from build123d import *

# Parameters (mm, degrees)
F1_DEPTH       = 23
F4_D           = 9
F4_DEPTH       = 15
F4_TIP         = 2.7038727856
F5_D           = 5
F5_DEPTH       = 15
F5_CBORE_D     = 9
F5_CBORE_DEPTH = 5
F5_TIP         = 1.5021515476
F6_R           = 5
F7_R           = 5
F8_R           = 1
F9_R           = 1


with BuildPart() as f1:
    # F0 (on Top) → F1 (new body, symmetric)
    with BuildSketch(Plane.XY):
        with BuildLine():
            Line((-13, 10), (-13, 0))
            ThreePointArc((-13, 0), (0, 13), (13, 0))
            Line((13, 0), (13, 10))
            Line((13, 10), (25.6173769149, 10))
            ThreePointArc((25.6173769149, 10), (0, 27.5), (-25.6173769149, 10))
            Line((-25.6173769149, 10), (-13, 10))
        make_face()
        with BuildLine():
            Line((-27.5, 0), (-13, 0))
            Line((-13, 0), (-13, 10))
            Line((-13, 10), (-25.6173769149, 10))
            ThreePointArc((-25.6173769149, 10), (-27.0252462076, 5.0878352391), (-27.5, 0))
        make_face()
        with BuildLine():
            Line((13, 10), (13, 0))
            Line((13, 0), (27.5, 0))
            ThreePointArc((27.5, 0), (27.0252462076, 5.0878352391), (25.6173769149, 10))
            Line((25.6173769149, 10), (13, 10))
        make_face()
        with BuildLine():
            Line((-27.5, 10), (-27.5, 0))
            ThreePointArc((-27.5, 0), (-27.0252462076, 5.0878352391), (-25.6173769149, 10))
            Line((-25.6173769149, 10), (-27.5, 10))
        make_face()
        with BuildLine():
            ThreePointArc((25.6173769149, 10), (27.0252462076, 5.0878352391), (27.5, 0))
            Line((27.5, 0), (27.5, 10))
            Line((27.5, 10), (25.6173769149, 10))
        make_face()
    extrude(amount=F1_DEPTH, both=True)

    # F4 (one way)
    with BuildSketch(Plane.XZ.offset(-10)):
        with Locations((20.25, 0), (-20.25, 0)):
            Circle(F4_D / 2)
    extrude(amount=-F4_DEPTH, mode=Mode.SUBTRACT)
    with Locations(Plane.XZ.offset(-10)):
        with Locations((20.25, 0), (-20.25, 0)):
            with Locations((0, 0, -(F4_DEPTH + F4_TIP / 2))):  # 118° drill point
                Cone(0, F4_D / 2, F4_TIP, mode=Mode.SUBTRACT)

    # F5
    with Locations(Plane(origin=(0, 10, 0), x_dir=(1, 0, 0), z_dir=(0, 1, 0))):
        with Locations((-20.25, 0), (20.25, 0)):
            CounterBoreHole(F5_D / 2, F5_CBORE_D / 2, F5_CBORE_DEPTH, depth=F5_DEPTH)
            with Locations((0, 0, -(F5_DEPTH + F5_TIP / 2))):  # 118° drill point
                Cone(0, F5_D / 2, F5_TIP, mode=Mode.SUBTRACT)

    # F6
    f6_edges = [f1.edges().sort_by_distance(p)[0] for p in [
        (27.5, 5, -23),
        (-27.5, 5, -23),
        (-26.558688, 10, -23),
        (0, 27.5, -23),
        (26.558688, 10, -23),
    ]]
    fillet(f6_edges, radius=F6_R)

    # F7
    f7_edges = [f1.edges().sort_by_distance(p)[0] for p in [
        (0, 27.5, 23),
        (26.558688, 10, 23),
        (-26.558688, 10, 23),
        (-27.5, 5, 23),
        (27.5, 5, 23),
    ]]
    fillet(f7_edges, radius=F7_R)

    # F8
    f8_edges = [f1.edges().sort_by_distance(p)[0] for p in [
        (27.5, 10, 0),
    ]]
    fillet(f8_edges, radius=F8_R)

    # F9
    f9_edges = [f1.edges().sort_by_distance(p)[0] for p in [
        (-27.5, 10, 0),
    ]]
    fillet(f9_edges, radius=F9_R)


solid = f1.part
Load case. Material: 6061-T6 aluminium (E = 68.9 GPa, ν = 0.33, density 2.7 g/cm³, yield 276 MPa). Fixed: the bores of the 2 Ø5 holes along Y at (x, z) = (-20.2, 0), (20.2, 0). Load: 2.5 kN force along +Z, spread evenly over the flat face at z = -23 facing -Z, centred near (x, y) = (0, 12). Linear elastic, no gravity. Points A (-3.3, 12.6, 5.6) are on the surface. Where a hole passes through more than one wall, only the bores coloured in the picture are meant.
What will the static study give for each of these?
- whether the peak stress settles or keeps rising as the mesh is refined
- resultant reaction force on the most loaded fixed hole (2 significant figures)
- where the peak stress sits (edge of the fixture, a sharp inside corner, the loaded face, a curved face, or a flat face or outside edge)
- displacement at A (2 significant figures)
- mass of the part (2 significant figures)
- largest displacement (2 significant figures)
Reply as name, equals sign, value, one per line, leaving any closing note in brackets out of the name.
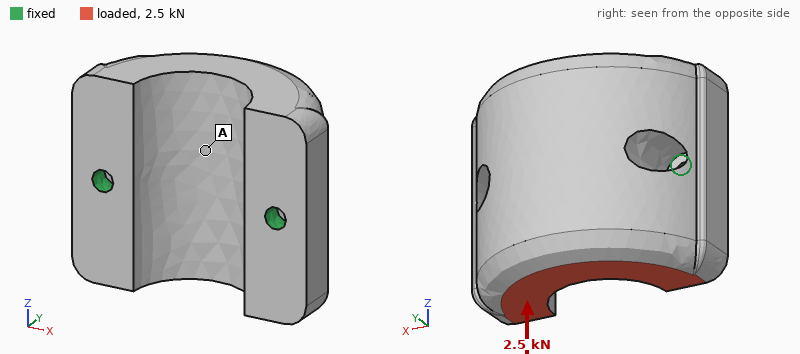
whether the peak stress settles or keeps rising as the mesh is refined = keeps rising
resultant reaction force on the most loaded fixed hole = 1.3 kN
where the peak stress sits = edge of the fixture
displacement at A = 19 µm
mass of the part = 110 g
largest displacement = 50 µm
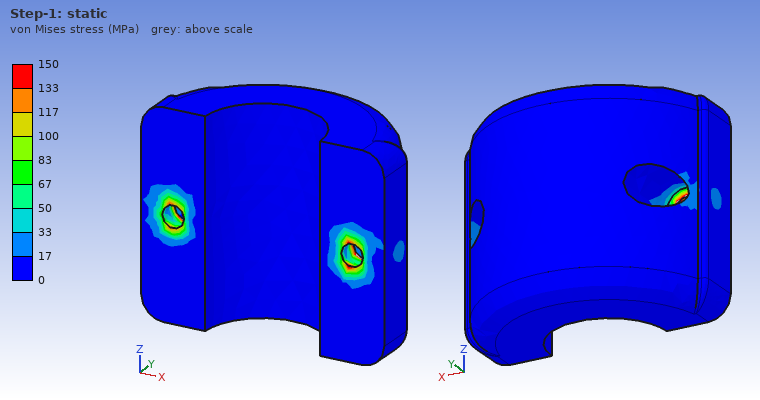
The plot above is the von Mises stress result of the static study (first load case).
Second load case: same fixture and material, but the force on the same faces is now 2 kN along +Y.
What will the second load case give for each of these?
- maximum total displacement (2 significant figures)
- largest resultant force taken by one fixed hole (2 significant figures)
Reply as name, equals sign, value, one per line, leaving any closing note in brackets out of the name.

maximum total displacement = 0.10 mm
largest resultant force taken by one fixed hole = 1.1 kN
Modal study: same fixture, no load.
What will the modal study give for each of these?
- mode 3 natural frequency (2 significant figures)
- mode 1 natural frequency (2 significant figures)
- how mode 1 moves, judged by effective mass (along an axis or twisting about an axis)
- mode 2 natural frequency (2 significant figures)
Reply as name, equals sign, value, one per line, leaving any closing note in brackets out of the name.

mode 3 natural frequency = 12 kHz
mode 1 natural frequency = 3200 Hz
how mode 1 moves, judged by effective mass = along Z
mode 2 natural frequency = 11 kHz
